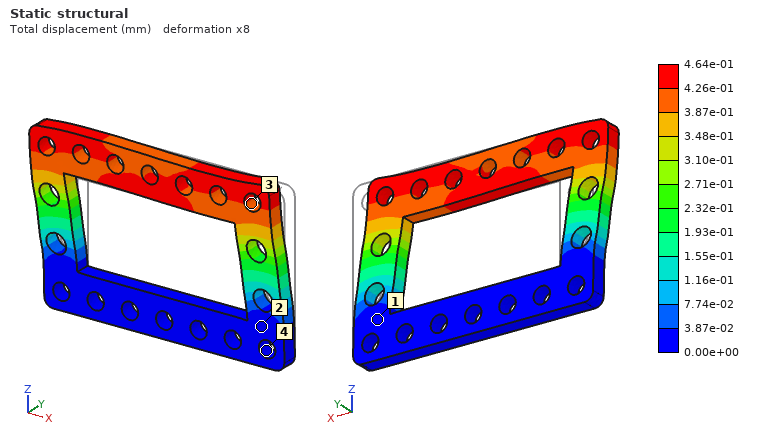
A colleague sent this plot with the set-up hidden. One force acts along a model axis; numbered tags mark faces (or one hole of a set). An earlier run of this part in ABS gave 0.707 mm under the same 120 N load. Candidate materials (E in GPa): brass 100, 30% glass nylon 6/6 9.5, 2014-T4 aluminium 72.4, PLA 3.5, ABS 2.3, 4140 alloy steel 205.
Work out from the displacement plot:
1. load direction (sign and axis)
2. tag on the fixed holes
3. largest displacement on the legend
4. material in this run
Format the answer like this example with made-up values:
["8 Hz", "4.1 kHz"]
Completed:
["-X", "4", "4.64e-01 mm", "PLA"]
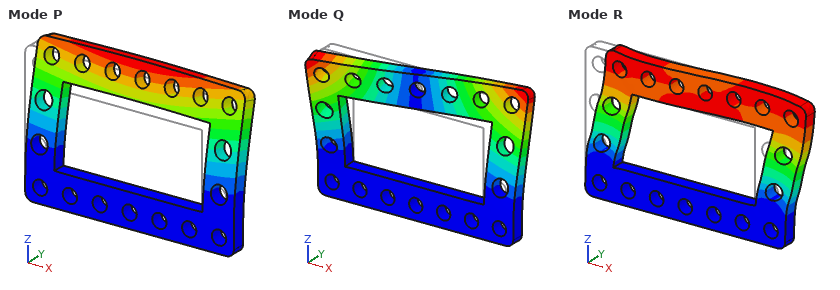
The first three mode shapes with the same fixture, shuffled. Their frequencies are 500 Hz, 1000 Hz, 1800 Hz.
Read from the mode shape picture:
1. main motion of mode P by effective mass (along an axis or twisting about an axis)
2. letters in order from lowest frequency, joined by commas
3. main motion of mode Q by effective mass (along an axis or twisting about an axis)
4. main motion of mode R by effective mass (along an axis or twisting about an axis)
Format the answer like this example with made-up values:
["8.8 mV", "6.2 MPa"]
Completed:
["along Y", "P, Q, R", "twisting about Z", "along X"]
